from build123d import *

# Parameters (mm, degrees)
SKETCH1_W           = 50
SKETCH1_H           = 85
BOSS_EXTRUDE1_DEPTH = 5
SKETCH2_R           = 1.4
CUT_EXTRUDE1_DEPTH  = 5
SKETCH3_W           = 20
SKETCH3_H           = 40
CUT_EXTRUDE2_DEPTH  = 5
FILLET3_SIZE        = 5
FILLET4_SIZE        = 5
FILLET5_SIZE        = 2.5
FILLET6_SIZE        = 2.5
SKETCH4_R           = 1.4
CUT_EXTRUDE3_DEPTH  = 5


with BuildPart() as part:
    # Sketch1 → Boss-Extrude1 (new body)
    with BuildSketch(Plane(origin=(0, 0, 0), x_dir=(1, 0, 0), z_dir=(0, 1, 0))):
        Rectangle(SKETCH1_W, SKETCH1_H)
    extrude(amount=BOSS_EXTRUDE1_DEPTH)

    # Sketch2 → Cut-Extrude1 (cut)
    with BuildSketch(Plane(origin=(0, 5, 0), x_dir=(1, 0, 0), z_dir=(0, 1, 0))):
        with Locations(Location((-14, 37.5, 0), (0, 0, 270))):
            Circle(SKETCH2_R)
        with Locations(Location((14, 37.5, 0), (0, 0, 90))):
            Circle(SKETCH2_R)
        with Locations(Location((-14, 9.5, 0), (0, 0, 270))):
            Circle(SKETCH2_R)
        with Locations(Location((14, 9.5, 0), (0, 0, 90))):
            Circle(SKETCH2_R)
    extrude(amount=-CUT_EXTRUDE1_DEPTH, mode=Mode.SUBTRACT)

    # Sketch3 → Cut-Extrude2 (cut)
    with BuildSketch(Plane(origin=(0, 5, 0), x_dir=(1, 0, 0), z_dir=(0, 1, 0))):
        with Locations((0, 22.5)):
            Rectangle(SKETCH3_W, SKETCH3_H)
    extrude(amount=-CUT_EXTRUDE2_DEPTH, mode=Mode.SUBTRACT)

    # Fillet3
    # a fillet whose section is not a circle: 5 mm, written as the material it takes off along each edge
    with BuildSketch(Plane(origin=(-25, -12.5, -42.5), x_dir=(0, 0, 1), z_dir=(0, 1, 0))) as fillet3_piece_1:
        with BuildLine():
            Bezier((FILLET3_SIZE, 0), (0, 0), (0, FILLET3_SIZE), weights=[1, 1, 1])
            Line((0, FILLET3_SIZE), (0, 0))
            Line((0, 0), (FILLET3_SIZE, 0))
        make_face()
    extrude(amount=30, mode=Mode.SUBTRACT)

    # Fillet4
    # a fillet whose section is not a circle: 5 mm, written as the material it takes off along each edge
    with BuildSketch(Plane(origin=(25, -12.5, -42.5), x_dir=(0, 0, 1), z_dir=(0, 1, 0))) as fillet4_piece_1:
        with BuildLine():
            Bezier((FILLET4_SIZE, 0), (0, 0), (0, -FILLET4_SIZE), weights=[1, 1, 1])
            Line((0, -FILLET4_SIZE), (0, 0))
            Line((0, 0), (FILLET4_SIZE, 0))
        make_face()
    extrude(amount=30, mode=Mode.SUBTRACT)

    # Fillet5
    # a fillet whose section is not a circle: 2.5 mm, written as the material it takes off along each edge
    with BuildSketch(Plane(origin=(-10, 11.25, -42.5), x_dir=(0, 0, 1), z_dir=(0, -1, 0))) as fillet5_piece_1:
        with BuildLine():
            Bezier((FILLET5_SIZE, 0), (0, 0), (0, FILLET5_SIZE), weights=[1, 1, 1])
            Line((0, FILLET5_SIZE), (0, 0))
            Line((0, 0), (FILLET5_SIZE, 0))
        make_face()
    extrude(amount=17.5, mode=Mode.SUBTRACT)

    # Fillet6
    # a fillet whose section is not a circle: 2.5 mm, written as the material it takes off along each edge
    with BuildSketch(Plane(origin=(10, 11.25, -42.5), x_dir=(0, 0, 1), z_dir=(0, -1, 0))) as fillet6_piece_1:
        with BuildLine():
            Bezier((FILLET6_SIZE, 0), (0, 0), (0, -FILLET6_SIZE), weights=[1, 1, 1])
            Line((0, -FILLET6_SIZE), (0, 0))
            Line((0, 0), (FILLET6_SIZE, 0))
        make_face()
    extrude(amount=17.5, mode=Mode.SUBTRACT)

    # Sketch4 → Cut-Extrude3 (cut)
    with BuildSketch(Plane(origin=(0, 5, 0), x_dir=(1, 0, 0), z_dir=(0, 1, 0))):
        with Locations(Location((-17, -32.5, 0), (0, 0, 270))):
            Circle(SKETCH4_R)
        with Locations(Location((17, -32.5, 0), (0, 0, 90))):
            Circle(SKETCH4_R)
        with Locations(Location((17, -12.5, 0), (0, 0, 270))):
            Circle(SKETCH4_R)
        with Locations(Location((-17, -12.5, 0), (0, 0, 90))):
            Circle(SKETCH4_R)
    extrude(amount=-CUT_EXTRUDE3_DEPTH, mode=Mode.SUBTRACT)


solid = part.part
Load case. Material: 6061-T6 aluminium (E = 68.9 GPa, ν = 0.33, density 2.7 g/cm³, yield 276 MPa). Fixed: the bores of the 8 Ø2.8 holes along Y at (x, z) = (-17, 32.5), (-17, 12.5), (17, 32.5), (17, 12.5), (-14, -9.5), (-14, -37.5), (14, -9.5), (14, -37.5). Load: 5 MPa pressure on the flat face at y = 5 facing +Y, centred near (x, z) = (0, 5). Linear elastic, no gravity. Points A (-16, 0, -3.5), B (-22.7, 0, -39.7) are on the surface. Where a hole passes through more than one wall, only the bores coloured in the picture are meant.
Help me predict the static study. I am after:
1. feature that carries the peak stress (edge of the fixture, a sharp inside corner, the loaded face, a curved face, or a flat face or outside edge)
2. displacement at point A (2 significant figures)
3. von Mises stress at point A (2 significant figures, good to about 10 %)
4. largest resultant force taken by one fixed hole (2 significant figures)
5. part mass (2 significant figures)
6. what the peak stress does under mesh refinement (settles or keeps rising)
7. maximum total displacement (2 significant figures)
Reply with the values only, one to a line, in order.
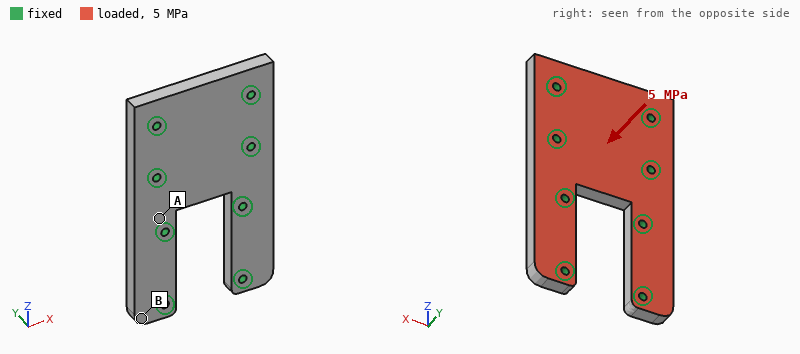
edge of the fixture
8.9 µm
55 MPa
2.5 kN
46 g
keeps rising
50 µm
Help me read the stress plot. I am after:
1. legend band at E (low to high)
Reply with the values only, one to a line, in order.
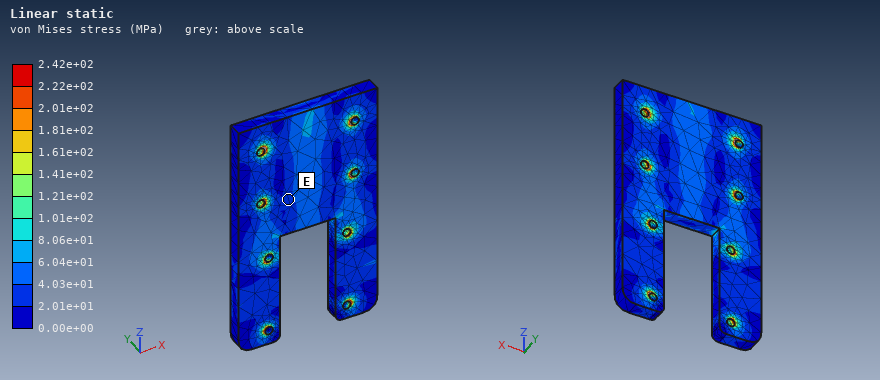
2.01e+01 to 4.03e+01 MPa
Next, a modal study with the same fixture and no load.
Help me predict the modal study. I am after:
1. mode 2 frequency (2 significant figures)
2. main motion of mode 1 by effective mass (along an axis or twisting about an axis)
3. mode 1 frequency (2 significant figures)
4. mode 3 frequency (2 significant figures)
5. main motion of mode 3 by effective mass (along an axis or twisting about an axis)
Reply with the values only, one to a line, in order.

19 kHz
along Y
17 kHz
20 kHz
twisting about Z
